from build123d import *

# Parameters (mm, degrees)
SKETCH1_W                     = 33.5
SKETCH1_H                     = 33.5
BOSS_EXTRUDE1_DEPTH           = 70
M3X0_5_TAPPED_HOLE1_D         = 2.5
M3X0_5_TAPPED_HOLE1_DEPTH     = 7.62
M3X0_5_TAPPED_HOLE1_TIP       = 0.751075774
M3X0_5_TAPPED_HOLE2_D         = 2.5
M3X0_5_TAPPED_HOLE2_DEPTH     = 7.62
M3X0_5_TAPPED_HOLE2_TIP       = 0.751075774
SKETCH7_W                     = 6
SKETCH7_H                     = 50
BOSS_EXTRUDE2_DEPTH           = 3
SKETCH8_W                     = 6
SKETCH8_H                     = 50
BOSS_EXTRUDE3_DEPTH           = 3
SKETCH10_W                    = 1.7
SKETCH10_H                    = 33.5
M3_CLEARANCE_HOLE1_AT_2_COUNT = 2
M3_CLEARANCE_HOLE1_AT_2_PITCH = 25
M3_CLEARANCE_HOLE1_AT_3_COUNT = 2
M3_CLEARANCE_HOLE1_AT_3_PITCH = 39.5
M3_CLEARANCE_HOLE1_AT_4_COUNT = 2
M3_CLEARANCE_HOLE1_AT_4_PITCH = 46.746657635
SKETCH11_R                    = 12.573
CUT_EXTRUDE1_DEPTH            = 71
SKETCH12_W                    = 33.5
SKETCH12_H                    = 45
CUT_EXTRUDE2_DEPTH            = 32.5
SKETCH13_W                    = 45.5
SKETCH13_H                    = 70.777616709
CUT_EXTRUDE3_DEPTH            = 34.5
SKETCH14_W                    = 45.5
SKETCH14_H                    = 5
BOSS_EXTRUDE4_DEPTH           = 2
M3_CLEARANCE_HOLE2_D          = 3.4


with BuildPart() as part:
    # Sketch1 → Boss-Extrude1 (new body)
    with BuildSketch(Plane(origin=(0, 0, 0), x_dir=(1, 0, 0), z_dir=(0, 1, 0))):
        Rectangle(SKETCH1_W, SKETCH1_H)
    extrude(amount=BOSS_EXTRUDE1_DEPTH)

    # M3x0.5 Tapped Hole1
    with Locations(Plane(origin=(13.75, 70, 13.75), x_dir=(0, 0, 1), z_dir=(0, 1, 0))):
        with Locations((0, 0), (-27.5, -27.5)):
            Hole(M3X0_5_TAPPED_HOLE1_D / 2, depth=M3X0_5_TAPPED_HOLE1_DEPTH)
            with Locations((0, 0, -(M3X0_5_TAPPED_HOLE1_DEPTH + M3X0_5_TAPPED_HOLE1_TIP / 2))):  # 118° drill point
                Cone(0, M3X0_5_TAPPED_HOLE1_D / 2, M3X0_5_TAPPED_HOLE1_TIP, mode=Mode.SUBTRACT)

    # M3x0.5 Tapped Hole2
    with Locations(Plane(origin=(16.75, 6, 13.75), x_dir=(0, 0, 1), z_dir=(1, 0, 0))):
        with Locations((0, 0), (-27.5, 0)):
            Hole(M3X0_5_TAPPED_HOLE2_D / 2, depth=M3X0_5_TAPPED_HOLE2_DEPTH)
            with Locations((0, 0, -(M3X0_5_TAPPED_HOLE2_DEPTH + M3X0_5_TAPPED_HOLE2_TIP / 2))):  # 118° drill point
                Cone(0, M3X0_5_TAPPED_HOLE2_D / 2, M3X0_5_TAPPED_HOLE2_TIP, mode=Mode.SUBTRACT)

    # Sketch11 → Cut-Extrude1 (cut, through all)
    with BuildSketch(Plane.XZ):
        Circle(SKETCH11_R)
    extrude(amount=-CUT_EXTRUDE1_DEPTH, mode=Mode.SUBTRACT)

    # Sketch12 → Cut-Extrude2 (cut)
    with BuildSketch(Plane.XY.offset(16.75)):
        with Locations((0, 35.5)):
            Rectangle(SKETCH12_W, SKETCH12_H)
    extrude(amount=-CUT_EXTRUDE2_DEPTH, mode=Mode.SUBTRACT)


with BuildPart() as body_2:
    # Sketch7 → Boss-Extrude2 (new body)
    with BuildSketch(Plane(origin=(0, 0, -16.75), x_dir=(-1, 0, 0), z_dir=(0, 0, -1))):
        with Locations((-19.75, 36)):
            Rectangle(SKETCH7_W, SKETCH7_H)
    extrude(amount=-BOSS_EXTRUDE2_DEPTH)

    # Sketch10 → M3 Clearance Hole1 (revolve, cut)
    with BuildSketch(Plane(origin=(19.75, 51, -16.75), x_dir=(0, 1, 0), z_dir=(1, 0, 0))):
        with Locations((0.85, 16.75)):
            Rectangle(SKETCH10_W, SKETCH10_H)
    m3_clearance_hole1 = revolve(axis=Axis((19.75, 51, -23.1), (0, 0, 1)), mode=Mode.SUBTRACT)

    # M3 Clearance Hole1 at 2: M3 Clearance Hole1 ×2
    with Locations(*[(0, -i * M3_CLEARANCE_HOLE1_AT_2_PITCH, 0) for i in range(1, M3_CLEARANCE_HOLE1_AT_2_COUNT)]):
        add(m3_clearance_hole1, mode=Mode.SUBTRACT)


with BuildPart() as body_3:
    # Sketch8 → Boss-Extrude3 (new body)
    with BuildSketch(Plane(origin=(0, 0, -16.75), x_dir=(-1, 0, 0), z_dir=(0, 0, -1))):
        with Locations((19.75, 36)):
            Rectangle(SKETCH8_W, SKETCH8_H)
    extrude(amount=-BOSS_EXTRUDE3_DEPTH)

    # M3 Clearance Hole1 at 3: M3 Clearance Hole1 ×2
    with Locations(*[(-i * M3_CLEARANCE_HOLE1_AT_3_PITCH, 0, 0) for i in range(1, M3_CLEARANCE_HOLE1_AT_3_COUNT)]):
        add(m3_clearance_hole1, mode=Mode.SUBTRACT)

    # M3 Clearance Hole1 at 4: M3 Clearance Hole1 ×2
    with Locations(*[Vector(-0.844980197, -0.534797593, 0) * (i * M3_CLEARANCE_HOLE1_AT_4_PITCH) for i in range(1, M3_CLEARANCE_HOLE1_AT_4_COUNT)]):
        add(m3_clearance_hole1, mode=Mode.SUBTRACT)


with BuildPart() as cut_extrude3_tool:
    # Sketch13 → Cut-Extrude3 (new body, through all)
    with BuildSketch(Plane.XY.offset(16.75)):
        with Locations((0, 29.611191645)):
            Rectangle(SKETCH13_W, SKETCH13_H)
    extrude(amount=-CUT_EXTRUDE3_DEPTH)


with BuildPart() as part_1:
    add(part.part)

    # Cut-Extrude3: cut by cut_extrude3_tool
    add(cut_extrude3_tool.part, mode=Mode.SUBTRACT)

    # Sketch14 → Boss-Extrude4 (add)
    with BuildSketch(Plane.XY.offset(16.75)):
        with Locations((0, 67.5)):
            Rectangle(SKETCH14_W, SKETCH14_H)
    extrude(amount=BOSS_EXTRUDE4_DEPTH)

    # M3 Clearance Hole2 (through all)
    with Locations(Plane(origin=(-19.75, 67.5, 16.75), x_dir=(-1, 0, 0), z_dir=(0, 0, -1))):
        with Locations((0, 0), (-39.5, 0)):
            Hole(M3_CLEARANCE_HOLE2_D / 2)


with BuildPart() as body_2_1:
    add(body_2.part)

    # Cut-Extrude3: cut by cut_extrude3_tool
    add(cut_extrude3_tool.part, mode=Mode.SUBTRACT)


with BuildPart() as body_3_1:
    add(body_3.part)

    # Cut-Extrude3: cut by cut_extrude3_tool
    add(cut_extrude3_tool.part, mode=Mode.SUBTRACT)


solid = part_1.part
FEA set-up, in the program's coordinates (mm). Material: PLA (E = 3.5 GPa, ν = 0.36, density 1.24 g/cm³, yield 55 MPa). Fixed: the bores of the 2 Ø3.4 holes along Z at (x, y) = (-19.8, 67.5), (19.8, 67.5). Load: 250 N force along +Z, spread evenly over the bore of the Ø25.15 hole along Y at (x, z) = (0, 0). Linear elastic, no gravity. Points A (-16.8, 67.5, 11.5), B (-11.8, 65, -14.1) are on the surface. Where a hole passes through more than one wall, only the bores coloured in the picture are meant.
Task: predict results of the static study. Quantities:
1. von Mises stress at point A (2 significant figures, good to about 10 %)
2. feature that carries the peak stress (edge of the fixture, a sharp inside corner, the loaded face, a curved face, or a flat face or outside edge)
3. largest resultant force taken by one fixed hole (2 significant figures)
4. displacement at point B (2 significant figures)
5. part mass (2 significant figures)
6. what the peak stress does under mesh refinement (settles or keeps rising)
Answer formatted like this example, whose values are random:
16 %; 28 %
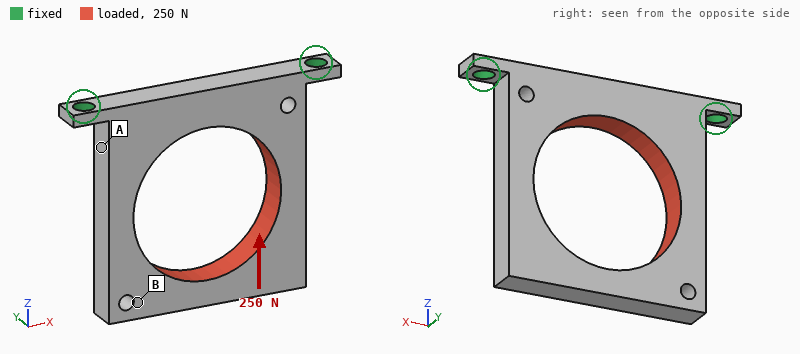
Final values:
7.9 MPa; edge of the fixture; 140 N; 0.081 mm; 4.3 g; keeps rising
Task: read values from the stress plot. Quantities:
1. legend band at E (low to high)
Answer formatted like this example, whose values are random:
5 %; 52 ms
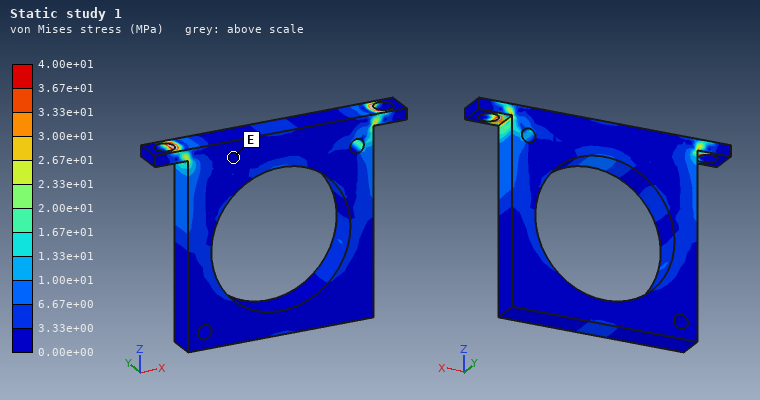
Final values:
0.00e+00 to 3.33e+00 MPa
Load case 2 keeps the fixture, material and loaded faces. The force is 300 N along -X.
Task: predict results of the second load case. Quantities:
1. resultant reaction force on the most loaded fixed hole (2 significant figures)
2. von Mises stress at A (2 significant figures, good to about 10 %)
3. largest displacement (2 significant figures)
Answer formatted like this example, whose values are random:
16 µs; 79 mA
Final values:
220 N; 17 MPa; 0.55 mm
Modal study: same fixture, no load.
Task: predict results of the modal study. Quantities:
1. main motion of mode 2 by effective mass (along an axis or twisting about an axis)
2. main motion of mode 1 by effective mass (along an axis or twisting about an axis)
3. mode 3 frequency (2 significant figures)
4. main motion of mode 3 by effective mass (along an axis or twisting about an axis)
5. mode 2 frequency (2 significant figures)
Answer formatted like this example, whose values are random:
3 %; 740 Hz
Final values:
twisting about Z; along Y; 2100 Hz; along X; 1500 Hz
